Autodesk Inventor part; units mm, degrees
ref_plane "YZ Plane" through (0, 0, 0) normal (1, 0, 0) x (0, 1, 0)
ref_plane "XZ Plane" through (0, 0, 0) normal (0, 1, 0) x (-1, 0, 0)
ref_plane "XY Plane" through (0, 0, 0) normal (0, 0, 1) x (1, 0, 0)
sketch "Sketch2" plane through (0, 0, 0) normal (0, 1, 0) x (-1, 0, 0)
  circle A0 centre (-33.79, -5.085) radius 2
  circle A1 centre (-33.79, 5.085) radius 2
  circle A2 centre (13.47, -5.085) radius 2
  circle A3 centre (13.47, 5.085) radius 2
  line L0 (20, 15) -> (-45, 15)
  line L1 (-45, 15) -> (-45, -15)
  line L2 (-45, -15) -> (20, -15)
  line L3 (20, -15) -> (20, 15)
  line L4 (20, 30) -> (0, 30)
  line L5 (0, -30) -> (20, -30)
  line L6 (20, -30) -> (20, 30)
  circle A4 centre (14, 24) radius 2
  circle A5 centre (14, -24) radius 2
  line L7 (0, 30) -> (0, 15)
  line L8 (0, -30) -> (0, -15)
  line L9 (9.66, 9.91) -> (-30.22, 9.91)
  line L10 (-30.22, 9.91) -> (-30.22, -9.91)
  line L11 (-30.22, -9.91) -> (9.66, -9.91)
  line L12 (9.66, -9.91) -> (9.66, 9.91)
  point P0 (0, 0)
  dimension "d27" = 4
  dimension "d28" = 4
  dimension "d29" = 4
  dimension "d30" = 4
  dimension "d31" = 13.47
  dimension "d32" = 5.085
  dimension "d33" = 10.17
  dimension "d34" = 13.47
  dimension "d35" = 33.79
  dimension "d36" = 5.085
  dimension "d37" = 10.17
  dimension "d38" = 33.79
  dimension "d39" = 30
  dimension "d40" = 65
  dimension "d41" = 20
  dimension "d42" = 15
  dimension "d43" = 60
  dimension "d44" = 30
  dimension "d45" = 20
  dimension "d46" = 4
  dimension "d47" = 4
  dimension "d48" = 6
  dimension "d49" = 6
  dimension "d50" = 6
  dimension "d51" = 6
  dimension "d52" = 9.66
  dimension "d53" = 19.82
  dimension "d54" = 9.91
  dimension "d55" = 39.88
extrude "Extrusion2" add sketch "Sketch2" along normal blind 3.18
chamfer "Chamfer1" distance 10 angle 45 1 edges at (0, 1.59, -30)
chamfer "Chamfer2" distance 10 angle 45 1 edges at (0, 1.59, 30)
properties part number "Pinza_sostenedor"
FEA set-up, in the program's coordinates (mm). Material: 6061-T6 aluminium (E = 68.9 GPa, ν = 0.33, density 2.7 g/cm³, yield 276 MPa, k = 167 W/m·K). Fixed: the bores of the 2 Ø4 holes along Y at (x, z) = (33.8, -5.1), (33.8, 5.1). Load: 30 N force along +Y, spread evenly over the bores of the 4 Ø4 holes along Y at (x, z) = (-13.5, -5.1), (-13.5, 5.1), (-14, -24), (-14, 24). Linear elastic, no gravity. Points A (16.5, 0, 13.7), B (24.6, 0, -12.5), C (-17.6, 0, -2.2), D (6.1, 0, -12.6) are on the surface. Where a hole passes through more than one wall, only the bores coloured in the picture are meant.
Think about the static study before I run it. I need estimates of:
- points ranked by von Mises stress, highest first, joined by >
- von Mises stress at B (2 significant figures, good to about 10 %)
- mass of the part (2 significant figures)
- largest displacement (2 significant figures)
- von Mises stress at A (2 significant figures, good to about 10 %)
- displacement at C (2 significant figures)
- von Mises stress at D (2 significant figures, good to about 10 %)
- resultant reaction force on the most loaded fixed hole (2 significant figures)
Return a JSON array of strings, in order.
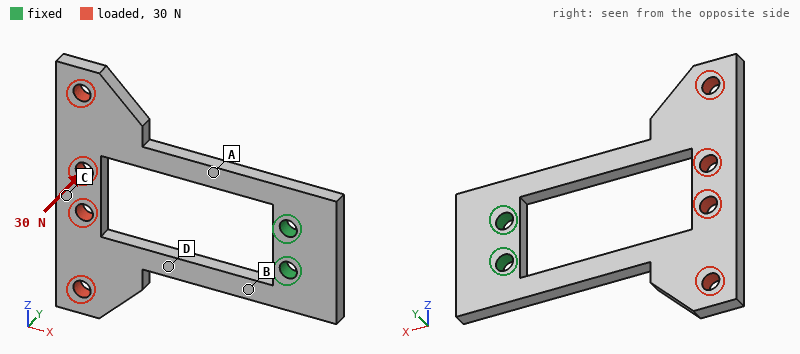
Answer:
["B > A > D > C", "67 MPa", "14 g", "0.72 mm", "53 MPa", "0.67 mm", "35 MPa", "15 N"]
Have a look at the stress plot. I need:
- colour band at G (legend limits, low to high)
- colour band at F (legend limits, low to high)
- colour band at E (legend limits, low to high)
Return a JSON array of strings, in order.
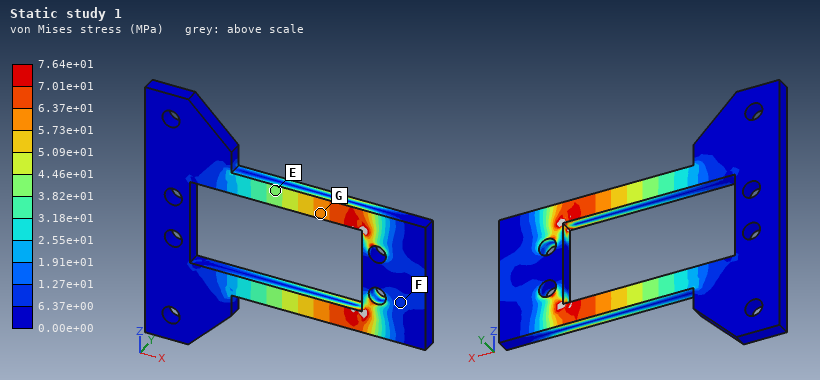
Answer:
["5.73e+01 to 6.37e+01 MPa", "6.37e+00 to 1.27e+01 MPa", "3.82e+01 to 4.46e+01 MPa"]
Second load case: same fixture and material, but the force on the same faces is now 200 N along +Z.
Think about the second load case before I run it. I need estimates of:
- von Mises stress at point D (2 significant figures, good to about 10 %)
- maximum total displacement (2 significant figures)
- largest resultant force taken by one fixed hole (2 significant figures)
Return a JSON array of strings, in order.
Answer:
["20 MPa", "0.31 mm", "570 N"]
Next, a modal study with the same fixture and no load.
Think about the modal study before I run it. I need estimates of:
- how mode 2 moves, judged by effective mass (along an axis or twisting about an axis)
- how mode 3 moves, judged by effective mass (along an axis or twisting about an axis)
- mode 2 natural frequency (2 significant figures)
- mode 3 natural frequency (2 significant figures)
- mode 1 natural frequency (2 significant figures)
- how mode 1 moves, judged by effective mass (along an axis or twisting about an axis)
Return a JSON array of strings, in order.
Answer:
["twisting about X", "along Z", "880 Hz", "1500 Hz", "430 Hz", "along Y"]
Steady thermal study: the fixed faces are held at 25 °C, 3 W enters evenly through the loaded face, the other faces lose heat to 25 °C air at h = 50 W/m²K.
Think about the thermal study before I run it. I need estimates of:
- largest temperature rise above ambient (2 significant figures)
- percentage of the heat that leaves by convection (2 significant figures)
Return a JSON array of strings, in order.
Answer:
["13 K", "53 %"]
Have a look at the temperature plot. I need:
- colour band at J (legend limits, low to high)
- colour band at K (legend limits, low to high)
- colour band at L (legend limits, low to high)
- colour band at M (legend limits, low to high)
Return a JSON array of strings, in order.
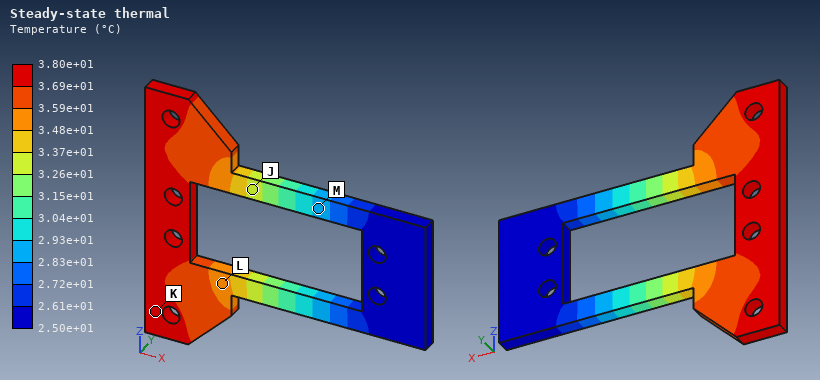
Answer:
["3.26e+01 to 3.37e+01 °C", "3.69e+01 to 3.80e+01 °C", "3.48e+01 to 3.59e+01 °C", "2.83e+01 to 2.93e+01 °C"]
